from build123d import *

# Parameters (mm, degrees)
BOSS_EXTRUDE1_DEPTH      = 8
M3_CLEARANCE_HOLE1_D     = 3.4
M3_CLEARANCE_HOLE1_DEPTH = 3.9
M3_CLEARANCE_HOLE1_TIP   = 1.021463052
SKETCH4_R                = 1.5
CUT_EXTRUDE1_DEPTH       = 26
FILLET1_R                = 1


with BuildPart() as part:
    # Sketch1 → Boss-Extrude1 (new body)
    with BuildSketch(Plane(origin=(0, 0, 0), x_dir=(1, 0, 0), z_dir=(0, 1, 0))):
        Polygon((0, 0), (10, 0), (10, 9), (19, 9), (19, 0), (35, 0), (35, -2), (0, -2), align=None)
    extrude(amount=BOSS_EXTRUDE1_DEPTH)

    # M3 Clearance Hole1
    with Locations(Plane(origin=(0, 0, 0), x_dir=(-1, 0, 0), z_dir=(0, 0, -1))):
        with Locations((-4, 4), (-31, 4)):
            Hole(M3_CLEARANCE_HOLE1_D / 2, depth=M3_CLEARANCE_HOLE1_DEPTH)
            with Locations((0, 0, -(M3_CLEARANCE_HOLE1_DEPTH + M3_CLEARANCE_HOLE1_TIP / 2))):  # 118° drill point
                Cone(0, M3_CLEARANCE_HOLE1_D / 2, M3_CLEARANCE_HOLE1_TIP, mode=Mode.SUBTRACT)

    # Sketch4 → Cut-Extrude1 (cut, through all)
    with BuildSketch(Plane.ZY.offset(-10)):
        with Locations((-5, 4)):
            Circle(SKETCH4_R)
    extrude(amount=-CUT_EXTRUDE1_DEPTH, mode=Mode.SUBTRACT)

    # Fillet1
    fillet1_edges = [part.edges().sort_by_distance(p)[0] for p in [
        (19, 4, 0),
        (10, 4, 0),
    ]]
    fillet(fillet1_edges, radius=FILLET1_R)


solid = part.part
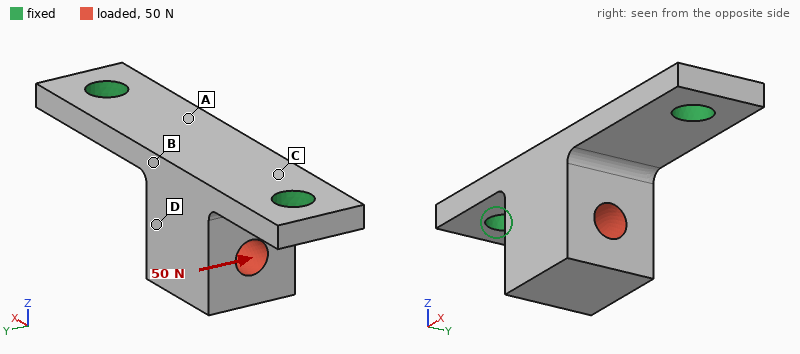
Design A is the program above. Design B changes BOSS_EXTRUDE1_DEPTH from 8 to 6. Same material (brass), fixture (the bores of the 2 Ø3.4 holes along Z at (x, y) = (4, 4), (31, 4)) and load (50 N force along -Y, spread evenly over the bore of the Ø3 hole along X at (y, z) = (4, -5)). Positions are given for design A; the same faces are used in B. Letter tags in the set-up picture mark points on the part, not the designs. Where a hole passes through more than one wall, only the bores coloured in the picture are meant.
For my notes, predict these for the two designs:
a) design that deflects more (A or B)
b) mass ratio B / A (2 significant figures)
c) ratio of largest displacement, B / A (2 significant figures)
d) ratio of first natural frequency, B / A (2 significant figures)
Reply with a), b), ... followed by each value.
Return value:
a) B
b) 0.73
c) 1.6
d) 0.96
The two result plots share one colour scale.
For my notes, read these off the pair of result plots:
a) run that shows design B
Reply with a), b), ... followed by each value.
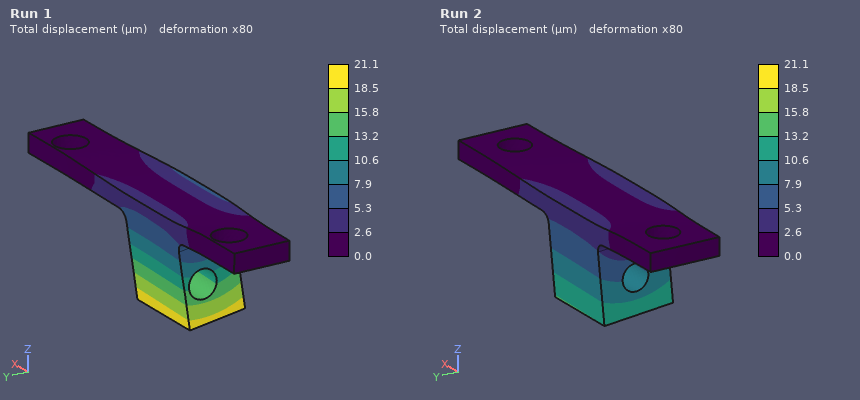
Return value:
a) Run 1
